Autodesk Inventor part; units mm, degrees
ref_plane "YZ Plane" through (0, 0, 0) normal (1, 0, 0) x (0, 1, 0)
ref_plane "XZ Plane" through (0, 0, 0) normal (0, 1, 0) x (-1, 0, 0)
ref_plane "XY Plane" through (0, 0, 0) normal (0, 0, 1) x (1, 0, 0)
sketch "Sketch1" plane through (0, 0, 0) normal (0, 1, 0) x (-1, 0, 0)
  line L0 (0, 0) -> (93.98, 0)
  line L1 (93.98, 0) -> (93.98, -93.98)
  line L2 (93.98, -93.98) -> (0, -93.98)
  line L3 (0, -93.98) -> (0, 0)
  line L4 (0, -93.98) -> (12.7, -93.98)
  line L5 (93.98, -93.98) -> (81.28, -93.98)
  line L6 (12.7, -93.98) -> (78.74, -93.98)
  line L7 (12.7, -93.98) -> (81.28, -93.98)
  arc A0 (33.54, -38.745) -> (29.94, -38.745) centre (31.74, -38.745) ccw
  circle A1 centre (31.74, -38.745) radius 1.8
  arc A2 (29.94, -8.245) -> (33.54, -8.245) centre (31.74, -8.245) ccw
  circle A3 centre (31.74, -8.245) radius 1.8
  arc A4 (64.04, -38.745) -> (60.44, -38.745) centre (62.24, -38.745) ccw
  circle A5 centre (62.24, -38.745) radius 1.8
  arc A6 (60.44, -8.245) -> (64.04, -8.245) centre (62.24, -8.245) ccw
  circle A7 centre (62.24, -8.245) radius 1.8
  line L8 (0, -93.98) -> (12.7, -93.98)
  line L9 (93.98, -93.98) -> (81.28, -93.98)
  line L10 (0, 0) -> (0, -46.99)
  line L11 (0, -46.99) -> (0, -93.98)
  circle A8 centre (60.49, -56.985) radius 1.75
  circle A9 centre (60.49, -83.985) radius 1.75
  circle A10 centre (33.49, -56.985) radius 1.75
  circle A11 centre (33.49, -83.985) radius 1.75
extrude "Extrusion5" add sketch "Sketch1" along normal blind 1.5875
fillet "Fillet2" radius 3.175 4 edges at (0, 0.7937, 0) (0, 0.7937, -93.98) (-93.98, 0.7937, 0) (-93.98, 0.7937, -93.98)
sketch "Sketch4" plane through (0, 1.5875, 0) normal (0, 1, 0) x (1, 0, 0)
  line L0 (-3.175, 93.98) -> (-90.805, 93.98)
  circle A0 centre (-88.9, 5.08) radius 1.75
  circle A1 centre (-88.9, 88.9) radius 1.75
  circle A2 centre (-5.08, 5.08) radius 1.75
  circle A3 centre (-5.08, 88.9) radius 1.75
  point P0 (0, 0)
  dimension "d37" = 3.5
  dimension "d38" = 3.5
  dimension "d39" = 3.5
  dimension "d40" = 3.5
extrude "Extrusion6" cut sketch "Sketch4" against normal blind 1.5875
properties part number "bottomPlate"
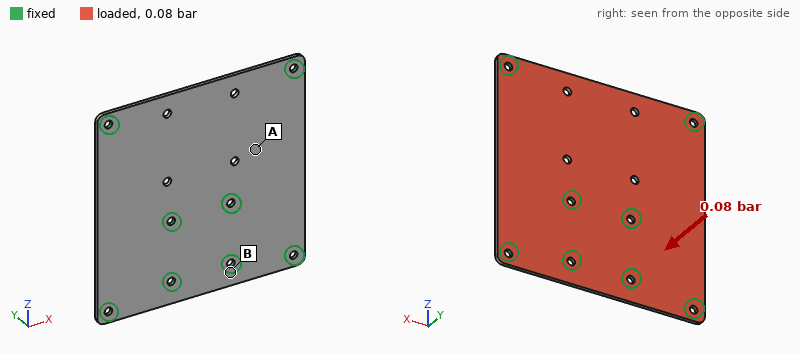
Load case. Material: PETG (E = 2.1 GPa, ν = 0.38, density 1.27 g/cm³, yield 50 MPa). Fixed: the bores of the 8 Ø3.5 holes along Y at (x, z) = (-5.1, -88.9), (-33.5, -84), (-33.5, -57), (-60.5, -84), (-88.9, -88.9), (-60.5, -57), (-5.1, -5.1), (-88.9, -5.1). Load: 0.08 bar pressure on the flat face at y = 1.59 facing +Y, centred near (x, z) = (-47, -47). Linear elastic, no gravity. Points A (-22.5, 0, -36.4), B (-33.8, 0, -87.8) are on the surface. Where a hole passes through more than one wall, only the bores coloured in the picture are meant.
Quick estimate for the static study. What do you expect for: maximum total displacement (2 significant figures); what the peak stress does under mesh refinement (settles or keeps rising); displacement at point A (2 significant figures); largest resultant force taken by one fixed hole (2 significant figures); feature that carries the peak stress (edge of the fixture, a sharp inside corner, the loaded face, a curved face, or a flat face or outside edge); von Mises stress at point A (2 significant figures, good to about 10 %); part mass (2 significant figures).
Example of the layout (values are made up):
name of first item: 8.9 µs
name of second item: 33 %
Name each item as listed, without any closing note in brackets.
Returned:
maximum total displacement: 1.3 mm
what the peak stress does under mesh refinement: keeps rising
displacement at point A: 0.51 mm
largest resultant force taken by one fixed hole: 15 N
feature that carries the peak stress: edge of the fixture
von Mises stress at point A: 3.4 MPa
part mass: 18 g
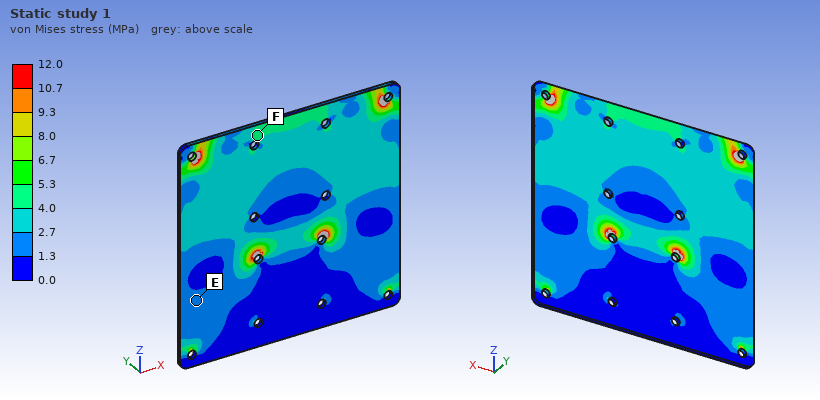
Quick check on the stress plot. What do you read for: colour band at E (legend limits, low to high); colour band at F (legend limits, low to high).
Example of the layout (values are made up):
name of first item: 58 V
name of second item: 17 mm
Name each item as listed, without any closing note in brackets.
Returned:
colour band at E: 1.3 to 2.7 MPa
colour band at F: 4.0 to 5.3 MPa
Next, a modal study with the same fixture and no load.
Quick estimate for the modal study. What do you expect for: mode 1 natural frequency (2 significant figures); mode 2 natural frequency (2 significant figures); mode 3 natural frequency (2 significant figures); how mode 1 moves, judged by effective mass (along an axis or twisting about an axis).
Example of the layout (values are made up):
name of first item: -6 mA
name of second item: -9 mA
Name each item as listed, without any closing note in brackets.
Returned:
mode 1 natural frequency: 350 Hz
mode 2 natural frequency: 470 Hz
mode 3 natural frequency: 480 Hz
how mode 1 moves, judged by effective mass: along Y
